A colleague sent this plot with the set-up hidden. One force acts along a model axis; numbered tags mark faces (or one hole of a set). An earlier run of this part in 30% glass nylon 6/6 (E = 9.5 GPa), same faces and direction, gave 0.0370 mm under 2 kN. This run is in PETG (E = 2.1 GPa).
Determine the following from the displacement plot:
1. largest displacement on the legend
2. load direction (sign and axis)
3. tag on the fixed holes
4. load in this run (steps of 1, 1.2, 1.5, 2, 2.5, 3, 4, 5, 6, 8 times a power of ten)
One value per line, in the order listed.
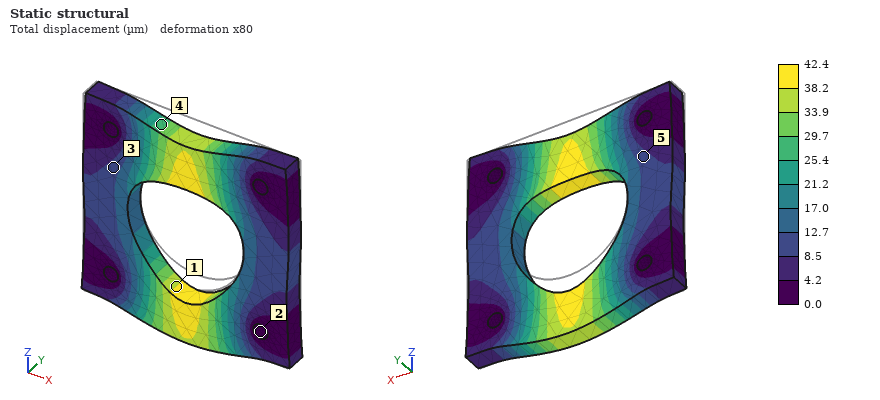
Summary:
42.4 µm
-Z
2
500 N
